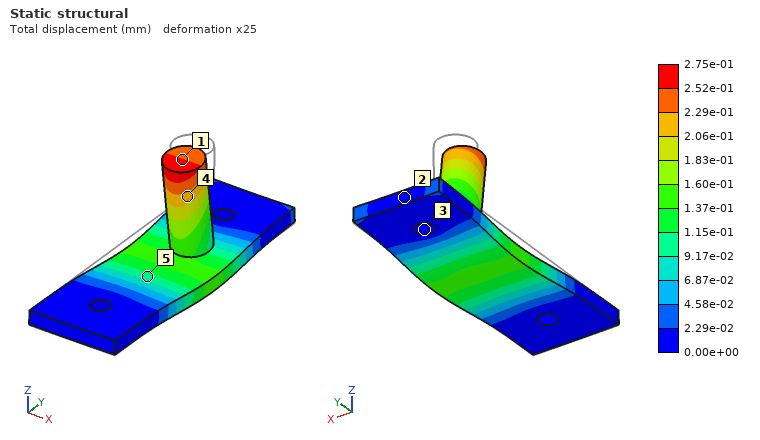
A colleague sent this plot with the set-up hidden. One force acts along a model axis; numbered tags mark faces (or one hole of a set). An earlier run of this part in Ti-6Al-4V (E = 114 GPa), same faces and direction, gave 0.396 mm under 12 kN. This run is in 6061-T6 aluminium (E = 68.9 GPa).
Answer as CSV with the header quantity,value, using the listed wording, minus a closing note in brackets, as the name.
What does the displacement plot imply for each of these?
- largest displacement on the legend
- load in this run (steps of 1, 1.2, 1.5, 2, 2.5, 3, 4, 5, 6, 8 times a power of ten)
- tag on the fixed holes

quantity,value
largest displacement on the legend,2.75e-01 mm
load in this run,5 kN
tag on the fixed holes,3
